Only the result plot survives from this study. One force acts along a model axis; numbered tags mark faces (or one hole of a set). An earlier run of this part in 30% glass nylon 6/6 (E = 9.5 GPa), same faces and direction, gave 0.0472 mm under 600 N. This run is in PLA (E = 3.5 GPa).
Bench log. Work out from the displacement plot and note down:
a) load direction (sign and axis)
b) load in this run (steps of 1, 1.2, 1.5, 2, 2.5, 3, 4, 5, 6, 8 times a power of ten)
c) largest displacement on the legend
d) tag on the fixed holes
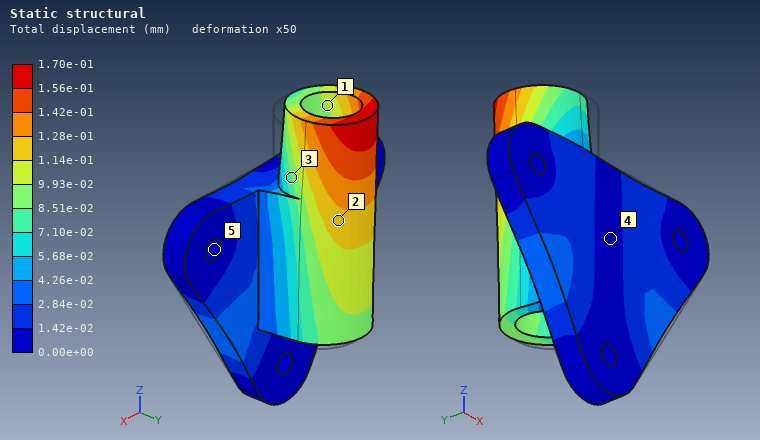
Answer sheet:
-X
800 N
1.70e-01 mm
5
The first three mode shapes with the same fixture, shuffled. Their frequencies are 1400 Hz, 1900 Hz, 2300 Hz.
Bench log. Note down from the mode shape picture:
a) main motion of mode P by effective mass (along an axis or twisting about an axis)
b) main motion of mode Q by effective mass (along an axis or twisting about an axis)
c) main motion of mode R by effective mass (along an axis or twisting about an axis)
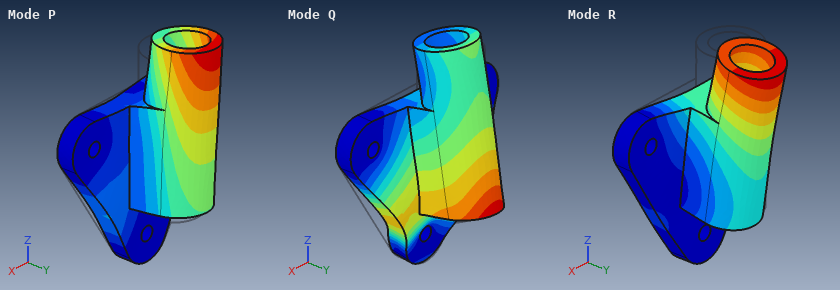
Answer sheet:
along X
along Y
along Y
